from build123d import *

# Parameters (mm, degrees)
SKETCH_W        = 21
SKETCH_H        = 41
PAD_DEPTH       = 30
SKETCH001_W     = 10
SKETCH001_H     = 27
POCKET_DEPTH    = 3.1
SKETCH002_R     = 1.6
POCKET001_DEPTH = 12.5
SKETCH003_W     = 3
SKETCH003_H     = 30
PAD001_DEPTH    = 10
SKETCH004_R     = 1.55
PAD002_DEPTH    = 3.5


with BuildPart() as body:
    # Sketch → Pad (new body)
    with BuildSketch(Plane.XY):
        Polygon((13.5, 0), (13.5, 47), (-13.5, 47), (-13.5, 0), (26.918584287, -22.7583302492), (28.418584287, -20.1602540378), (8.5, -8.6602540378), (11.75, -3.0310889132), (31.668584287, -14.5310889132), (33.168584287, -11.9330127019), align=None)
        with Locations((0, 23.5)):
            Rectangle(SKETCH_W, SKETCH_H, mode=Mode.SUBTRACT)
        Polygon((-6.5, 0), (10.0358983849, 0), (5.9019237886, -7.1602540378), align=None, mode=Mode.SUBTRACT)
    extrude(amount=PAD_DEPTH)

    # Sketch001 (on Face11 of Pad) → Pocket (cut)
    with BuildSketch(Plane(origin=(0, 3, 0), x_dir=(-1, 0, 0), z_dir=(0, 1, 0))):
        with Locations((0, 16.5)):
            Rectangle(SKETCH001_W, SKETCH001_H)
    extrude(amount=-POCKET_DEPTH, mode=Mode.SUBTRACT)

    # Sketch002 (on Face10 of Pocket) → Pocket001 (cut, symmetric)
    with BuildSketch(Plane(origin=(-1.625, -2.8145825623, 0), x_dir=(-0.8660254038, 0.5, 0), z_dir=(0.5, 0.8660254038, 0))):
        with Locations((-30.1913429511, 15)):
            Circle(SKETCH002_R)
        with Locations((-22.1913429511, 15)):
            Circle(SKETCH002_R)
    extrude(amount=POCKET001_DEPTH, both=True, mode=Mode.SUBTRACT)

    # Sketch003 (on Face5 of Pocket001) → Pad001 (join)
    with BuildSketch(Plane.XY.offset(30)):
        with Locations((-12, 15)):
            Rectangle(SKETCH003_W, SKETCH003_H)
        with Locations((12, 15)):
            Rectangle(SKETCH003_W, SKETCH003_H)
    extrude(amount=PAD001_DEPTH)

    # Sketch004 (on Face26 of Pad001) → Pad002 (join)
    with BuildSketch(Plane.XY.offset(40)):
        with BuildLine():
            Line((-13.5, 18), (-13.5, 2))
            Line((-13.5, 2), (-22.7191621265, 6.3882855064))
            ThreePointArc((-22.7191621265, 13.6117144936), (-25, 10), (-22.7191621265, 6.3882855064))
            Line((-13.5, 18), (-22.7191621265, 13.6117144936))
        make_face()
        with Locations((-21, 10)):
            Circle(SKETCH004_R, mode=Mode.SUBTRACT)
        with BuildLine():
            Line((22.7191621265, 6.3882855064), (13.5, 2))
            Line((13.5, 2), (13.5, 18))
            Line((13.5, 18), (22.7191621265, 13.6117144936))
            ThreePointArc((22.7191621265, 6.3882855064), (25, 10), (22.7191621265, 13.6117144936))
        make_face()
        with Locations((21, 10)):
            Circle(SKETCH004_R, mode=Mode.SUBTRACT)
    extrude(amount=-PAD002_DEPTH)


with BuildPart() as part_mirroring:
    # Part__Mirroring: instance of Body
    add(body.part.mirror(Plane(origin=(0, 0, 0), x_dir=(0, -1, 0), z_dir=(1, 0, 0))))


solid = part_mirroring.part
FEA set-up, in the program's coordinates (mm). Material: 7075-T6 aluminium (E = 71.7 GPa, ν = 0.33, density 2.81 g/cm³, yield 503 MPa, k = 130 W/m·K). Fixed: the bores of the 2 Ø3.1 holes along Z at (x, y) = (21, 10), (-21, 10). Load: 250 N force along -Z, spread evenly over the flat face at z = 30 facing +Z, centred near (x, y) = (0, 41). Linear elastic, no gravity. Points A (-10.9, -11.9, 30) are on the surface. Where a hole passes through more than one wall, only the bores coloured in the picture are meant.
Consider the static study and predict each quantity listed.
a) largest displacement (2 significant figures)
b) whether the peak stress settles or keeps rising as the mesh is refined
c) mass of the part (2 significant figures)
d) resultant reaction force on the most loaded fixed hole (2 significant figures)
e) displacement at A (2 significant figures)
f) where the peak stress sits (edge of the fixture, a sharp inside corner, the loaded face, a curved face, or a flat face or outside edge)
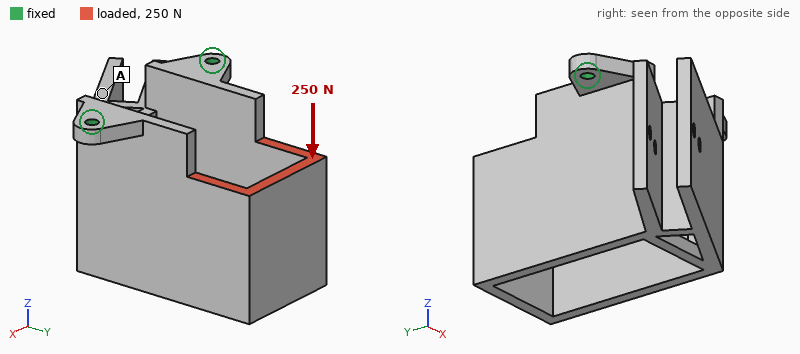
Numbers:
0.37 mm
keeps rising
60 g
130 N
0.15 mm
edge of the fixture
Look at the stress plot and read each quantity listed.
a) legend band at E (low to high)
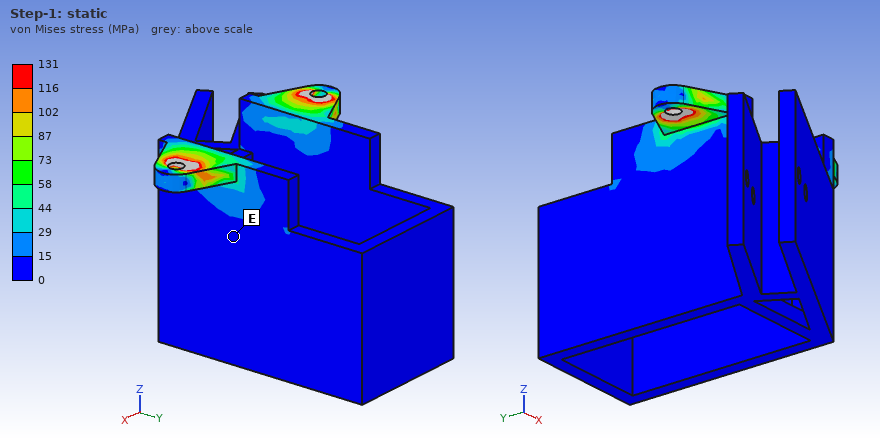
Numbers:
0 to 15 MPa
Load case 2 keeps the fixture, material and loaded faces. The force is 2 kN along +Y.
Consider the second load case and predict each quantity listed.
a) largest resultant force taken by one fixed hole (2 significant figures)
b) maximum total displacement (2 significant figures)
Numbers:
1.0 kN
0.81 mm
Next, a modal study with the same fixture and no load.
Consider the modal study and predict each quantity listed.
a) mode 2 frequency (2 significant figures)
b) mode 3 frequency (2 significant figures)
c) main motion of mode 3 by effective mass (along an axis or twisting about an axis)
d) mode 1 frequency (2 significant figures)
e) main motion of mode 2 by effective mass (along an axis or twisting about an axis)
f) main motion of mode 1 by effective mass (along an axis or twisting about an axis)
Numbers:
1700 Hz
2700 Hz
along X
710 Hz
along X
along Y
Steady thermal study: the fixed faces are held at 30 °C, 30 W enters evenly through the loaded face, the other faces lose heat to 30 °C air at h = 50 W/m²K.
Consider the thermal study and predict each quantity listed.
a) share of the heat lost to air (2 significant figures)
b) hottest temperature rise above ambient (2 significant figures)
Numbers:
54 %
57 K
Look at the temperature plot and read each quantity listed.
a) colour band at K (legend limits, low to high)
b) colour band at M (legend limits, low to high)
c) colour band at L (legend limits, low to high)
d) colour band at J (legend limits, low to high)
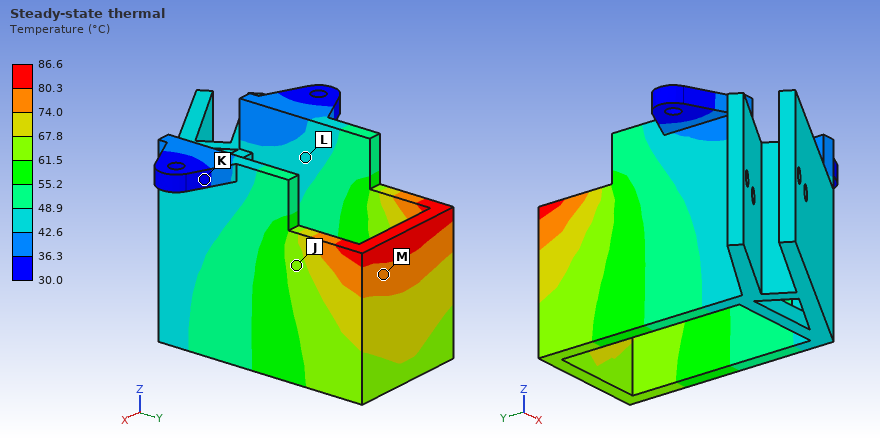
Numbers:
30.0 to 36.3 °C
74.0 to 80.3 °C
42.6 to 48.9 °C
61.5 to 67.8 °C
